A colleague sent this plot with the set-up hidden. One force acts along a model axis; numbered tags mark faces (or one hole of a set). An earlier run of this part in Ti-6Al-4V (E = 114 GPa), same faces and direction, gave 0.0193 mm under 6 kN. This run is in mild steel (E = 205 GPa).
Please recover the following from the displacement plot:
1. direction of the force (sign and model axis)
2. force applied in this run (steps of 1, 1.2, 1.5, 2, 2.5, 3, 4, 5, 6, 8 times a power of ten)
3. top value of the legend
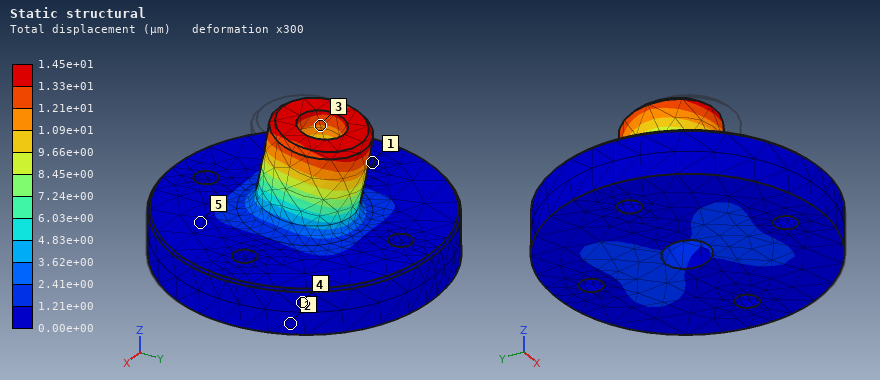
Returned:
+Y
8 kN
1.45e+01 µm
